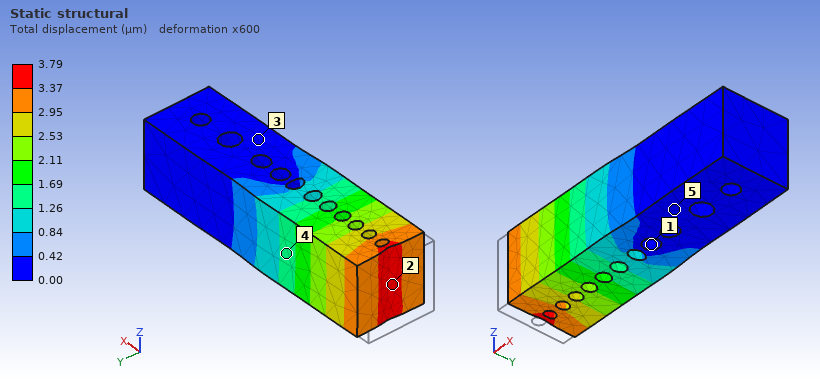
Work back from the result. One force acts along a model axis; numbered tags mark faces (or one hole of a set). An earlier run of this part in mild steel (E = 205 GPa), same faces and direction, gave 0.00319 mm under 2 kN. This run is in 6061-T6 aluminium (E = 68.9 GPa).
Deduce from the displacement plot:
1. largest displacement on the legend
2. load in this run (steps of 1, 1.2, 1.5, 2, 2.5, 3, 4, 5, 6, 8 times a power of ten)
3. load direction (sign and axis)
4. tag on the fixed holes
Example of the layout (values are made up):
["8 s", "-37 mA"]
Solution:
["3.79 µm", "800 N", "+X", "1"]
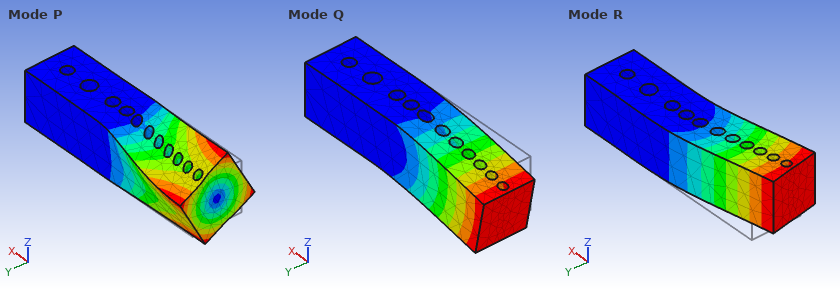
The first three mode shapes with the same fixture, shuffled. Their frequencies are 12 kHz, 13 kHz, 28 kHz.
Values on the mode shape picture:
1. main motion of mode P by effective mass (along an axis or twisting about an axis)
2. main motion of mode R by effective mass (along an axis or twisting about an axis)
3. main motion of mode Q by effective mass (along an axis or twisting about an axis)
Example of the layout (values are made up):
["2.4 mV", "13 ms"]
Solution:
["twisting about X", "along Y", "along Z"]
